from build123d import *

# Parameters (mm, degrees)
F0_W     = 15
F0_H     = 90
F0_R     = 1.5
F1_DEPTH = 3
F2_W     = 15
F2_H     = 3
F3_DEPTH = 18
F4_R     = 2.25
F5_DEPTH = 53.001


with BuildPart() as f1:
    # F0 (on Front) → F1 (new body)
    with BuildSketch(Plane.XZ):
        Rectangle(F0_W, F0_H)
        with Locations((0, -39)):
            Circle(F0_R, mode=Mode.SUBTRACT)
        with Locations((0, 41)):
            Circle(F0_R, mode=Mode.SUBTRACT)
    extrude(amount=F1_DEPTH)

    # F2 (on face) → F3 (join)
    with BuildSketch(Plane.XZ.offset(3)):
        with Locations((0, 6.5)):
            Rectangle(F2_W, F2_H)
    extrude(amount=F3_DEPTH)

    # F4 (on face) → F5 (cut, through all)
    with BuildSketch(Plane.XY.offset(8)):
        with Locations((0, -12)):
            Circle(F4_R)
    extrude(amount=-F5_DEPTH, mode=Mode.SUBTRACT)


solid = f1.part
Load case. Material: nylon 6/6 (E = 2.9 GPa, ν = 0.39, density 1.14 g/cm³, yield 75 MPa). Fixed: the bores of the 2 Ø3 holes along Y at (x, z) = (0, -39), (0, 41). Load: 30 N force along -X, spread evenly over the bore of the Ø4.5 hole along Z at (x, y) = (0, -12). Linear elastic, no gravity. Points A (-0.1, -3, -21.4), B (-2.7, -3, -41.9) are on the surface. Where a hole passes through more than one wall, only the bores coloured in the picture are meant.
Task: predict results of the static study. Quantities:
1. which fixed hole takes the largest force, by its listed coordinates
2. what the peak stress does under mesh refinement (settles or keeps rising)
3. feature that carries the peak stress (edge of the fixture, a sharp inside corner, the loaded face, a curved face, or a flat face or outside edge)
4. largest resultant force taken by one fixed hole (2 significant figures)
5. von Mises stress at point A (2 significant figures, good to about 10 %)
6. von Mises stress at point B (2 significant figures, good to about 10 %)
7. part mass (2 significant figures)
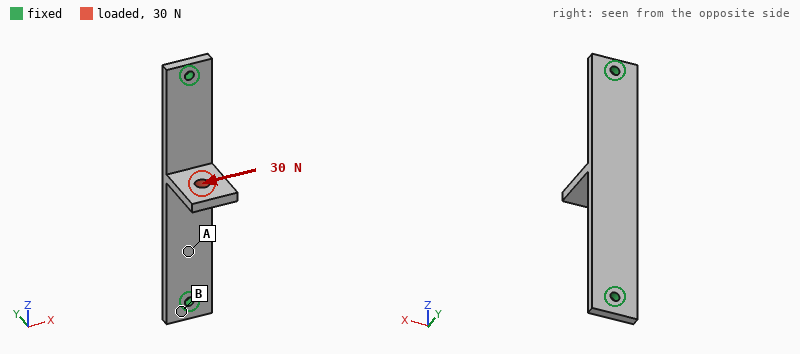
(0, 41)
keeps rising
edge of the fixture
17 N
6.6 MPa
1.8 MPa
5.4 g
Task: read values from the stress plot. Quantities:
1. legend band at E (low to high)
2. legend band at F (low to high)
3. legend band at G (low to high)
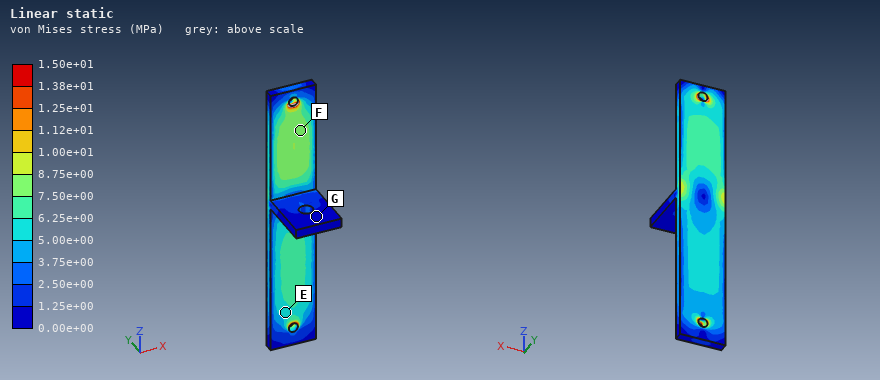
5.00e+00 to 6.25e+00 MPa
7.50e+00 to 8.75e+00 MPa
0.00e+00 to 1.25e+00 MPa
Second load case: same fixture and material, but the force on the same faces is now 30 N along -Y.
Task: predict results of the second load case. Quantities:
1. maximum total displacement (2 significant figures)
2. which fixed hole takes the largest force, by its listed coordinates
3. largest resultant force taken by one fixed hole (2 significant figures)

0.76 mm
(0, 41)
18 N
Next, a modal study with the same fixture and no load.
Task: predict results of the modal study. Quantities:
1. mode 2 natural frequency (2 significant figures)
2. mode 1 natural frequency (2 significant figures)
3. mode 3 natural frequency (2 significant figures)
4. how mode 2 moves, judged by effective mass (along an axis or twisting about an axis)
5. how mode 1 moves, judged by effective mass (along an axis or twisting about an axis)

990 Hz
640 Hz
1400 Hz
along X
along Y
